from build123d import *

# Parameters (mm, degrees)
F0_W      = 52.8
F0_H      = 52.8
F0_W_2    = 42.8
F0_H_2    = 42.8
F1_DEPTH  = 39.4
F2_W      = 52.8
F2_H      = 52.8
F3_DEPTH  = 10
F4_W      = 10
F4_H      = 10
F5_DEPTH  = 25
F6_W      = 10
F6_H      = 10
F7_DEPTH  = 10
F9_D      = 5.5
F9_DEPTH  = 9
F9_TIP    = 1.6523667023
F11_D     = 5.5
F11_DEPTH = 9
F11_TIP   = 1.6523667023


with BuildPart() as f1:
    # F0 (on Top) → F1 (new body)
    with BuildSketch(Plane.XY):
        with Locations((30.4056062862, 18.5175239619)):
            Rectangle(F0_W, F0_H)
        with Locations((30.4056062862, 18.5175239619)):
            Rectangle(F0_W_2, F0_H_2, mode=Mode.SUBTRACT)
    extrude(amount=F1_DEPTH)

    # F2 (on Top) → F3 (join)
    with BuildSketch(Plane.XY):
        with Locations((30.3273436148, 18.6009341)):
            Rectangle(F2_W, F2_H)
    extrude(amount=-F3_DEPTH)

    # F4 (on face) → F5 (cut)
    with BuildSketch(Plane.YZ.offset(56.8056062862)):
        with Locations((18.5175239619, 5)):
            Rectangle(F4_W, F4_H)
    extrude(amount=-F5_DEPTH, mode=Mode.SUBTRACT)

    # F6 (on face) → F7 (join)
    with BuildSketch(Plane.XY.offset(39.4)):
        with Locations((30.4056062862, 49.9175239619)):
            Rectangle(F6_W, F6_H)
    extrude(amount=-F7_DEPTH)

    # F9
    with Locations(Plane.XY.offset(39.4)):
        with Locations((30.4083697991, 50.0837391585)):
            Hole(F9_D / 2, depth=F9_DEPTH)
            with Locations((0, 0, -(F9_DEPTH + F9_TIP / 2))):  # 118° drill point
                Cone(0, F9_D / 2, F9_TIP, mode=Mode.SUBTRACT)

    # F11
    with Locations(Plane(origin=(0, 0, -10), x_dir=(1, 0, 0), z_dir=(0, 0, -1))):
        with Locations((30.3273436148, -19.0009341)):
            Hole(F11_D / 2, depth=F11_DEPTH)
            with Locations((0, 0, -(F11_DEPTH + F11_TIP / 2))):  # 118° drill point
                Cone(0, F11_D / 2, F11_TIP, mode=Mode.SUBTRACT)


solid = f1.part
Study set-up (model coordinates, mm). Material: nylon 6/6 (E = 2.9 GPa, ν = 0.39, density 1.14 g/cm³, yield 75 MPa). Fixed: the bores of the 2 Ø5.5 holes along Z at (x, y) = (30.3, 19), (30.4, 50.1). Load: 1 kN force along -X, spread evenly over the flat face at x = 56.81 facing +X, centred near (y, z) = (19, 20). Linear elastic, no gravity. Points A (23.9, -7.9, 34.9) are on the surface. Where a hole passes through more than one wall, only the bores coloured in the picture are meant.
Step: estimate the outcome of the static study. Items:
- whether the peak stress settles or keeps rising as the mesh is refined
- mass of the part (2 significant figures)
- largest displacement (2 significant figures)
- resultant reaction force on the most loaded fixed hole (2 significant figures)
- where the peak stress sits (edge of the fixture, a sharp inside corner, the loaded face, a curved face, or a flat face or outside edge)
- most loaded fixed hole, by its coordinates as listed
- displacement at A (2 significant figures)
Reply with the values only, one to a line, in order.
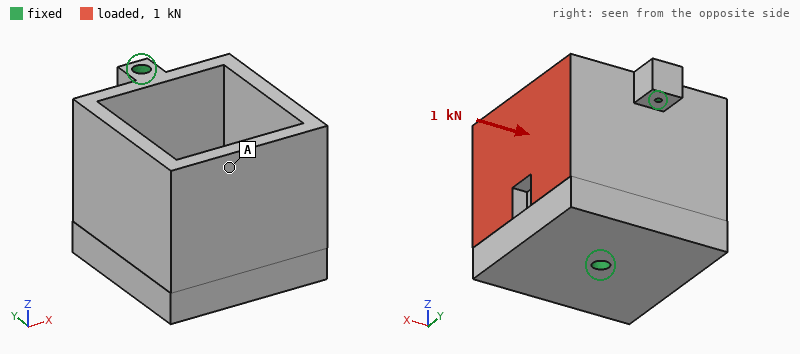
keeps rising
75 g
1.1 mm
660 N
edge of the fixture
(30.3, 19)
0.85 mm
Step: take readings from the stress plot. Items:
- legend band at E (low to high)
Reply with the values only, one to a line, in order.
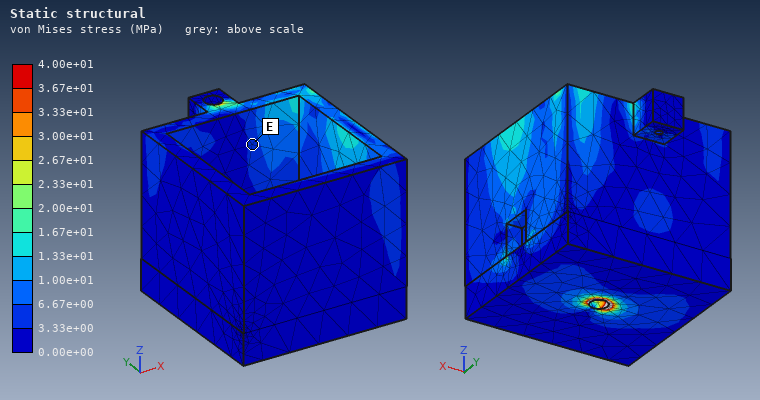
3.33e+00 to 6.67e+00 MPa
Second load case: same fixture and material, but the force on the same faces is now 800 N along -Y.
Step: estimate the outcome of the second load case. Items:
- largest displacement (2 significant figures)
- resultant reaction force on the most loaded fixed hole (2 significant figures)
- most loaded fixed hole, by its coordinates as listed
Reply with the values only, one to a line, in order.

0.93 mm
740 N
(30.3, 19)
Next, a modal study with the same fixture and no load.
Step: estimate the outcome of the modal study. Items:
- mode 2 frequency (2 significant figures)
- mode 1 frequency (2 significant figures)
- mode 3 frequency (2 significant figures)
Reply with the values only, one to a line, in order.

1300 Hz
740 Hz
1300 Hz
